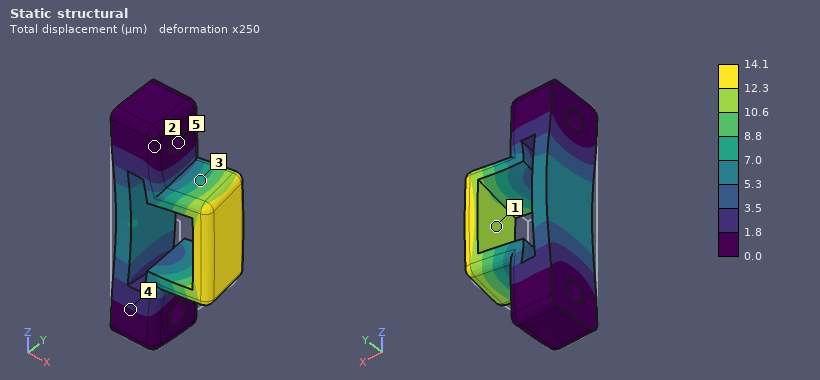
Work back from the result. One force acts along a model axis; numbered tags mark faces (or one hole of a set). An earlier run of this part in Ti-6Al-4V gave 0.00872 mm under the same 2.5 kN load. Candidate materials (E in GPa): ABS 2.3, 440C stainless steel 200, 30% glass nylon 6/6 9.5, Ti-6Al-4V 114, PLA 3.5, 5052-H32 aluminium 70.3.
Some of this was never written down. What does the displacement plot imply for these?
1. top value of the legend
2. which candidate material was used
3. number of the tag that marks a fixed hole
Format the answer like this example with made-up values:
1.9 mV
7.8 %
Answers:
14.1 µm
5052-H32 aluminium
5
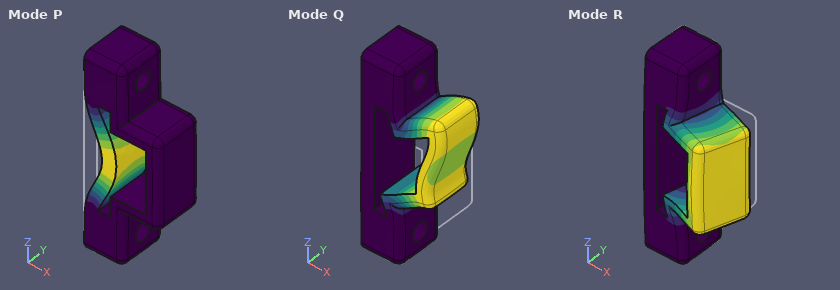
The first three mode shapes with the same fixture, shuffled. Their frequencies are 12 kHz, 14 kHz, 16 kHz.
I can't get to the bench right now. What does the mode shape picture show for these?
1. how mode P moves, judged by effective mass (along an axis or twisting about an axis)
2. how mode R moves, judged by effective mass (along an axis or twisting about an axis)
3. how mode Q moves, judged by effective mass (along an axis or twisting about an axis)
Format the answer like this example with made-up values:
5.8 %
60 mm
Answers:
along X
along Y
along Z
